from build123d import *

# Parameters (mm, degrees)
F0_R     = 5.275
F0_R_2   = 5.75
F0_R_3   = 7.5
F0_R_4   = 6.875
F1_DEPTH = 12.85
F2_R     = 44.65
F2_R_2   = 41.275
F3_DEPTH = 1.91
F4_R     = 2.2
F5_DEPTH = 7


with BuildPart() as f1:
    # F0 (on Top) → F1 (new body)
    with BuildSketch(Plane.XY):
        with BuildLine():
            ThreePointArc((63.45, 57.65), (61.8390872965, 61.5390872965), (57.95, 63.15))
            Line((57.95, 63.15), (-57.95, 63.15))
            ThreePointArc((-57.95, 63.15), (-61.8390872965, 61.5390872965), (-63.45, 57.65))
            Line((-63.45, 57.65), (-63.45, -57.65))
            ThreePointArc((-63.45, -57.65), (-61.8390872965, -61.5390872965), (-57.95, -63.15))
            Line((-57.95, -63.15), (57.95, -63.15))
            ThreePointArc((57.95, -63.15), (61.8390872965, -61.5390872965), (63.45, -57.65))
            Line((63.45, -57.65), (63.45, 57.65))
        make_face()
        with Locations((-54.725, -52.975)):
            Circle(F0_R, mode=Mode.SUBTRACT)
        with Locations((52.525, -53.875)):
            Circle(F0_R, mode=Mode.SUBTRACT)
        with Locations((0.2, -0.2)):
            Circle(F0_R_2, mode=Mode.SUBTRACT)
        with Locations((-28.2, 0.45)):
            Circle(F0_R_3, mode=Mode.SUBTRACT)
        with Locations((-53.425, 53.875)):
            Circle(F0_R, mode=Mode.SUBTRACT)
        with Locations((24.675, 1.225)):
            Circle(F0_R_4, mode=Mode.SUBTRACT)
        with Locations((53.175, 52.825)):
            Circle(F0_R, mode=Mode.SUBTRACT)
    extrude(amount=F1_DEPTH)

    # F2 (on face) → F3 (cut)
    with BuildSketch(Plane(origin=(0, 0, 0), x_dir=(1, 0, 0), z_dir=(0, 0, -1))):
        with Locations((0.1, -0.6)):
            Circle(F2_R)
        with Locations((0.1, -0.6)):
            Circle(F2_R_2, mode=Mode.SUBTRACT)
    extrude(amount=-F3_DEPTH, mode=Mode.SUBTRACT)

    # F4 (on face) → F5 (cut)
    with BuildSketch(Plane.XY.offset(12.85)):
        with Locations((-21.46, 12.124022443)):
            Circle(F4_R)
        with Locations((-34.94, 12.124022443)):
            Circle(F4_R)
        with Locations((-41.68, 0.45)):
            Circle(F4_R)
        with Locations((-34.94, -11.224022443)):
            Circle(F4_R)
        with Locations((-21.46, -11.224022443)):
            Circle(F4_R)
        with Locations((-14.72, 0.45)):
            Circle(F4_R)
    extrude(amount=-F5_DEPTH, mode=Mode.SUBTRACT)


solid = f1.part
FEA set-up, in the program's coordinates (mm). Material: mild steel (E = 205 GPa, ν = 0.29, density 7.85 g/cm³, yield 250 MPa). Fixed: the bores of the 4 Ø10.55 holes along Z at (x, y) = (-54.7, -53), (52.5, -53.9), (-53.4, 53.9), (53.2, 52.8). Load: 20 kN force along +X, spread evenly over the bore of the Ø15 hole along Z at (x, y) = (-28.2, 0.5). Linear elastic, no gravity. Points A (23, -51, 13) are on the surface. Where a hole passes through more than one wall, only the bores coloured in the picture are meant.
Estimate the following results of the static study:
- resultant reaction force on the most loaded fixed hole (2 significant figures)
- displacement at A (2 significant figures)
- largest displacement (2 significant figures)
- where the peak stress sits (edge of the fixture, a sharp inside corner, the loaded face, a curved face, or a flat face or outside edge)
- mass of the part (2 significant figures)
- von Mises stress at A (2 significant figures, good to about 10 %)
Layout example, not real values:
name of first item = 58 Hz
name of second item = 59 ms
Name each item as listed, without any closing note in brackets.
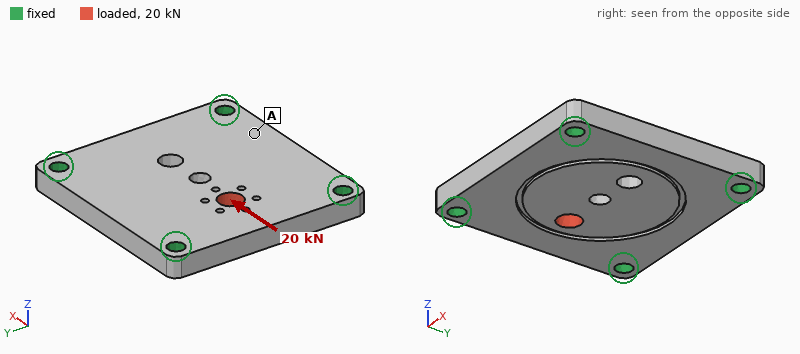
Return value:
resultant reaction force on the most loaded fixed hole = 6.1 kN
displacement at A = 1.6 µm
largest displacement = 10 µm
where the peak stress sits = a curved face
mass of the part = 1.5 kg
von Mises stress at A = 8.9 MPa
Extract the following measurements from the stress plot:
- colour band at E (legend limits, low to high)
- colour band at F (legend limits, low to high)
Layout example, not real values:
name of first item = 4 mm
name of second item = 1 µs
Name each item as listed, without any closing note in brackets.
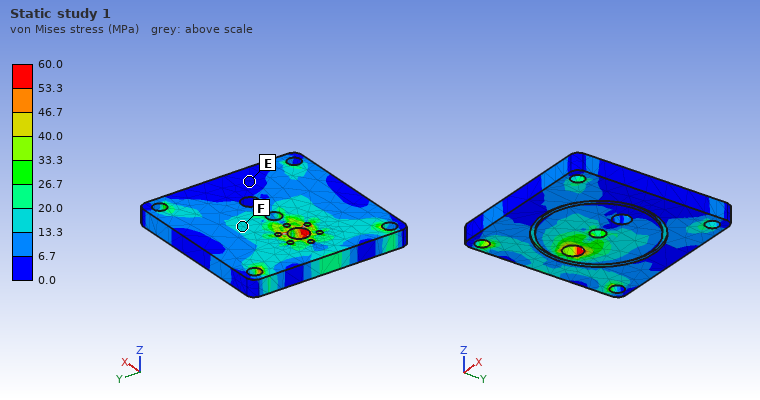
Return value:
colour band at E = 0.0 to 6.7 MPa
colour band at F = 13.3 to 20.0 MPa
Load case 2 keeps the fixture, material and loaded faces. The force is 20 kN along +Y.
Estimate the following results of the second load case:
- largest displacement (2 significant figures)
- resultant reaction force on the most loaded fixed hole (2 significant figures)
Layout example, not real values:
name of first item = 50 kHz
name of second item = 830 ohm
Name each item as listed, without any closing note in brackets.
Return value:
largest displacement = 7.2 µm
resultant reaction force on the most loaded fixed hole = 7.7 kN
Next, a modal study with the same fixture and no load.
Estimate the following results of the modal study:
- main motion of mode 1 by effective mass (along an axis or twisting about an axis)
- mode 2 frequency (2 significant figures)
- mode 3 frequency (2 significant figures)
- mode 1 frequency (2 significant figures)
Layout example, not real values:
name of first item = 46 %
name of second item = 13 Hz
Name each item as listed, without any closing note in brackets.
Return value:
main motion of mode 1 by effective mass = along Z
mode 2 frequency = 6200 Hz
mode 3 frequency = 6300 Hz
mode 1 frequency = 3700 Hz
